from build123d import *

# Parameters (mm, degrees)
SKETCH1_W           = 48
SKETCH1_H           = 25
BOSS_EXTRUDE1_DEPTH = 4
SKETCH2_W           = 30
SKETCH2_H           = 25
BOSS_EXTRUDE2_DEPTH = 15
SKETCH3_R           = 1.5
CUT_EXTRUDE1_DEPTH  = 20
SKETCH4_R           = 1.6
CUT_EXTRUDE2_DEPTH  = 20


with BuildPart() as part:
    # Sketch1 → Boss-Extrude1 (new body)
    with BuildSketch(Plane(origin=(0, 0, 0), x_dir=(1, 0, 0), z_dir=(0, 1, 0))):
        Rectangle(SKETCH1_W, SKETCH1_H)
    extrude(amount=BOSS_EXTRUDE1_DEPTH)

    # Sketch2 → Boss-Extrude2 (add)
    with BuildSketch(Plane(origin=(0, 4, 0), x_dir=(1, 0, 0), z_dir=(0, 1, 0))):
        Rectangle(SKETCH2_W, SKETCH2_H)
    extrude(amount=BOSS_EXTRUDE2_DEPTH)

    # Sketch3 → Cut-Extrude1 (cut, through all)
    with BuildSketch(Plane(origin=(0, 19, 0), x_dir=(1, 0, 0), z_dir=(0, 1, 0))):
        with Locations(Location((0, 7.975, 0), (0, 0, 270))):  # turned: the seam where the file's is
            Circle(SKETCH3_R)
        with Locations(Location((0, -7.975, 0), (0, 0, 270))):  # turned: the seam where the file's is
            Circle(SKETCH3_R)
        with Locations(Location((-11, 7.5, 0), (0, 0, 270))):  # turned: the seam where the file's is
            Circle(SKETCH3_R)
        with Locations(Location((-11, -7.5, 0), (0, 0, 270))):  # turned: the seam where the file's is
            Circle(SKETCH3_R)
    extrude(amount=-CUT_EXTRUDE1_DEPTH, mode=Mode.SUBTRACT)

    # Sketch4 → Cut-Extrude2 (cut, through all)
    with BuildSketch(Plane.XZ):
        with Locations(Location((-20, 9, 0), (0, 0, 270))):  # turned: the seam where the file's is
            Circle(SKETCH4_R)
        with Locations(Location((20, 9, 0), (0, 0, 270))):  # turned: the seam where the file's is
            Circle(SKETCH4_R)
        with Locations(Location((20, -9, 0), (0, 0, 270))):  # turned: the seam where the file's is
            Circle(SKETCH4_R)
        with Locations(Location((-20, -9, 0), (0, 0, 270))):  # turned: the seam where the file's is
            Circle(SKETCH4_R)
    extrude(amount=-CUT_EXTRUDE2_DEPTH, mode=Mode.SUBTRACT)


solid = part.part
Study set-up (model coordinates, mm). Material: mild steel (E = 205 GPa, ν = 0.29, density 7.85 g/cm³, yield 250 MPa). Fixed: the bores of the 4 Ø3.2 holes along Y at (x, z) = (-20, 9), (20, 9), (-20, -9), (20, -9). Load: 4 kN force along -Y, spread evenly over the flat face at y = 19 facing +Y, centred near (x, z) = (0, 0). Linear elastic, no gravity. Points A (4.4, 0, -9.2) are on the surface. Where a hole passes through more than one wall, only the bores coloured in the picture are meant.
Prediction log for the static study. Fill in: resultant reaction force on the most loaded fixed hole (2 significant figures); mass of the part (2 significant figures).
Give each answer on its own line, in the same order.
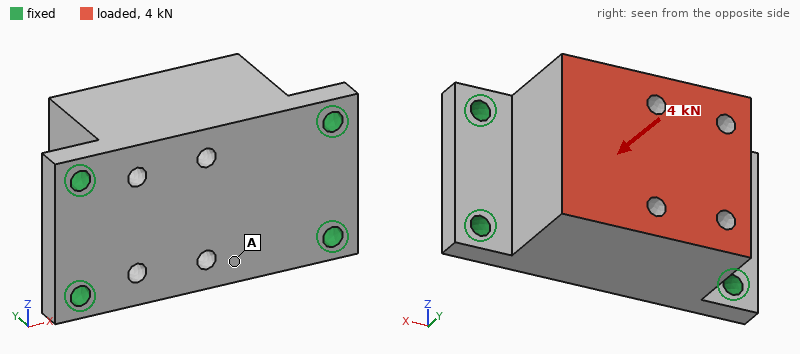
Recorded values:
1.1 kN
120 g
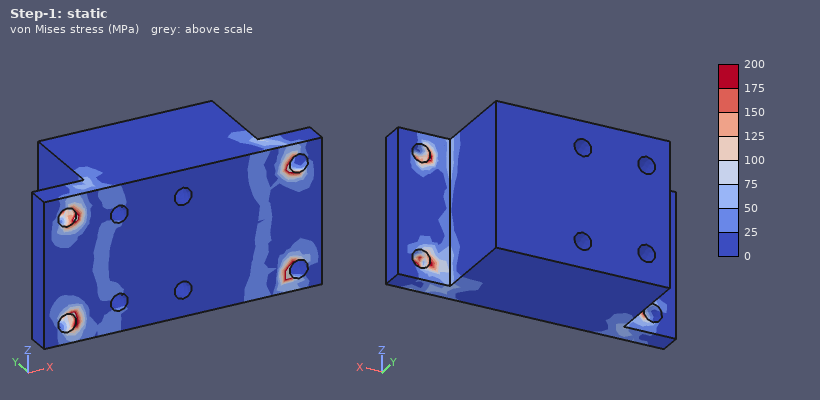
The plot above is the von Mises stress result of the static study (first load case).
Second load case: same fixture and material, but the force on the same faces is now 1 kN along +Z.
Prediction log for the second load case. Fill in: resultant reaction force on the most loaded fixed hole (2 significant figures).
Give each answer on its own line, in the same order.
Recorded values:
610 N
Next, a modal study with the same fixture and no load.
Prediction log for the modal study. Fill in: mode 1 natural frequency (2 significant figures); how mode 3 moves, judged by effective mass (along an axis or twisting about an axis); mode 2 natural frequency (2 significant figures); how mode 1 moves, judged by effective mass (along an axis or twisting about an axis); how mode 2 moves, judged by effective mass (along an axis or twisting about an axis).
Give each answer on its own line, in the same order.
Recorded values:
9900 Hz
along X
14 kHz
along Z
along Y
